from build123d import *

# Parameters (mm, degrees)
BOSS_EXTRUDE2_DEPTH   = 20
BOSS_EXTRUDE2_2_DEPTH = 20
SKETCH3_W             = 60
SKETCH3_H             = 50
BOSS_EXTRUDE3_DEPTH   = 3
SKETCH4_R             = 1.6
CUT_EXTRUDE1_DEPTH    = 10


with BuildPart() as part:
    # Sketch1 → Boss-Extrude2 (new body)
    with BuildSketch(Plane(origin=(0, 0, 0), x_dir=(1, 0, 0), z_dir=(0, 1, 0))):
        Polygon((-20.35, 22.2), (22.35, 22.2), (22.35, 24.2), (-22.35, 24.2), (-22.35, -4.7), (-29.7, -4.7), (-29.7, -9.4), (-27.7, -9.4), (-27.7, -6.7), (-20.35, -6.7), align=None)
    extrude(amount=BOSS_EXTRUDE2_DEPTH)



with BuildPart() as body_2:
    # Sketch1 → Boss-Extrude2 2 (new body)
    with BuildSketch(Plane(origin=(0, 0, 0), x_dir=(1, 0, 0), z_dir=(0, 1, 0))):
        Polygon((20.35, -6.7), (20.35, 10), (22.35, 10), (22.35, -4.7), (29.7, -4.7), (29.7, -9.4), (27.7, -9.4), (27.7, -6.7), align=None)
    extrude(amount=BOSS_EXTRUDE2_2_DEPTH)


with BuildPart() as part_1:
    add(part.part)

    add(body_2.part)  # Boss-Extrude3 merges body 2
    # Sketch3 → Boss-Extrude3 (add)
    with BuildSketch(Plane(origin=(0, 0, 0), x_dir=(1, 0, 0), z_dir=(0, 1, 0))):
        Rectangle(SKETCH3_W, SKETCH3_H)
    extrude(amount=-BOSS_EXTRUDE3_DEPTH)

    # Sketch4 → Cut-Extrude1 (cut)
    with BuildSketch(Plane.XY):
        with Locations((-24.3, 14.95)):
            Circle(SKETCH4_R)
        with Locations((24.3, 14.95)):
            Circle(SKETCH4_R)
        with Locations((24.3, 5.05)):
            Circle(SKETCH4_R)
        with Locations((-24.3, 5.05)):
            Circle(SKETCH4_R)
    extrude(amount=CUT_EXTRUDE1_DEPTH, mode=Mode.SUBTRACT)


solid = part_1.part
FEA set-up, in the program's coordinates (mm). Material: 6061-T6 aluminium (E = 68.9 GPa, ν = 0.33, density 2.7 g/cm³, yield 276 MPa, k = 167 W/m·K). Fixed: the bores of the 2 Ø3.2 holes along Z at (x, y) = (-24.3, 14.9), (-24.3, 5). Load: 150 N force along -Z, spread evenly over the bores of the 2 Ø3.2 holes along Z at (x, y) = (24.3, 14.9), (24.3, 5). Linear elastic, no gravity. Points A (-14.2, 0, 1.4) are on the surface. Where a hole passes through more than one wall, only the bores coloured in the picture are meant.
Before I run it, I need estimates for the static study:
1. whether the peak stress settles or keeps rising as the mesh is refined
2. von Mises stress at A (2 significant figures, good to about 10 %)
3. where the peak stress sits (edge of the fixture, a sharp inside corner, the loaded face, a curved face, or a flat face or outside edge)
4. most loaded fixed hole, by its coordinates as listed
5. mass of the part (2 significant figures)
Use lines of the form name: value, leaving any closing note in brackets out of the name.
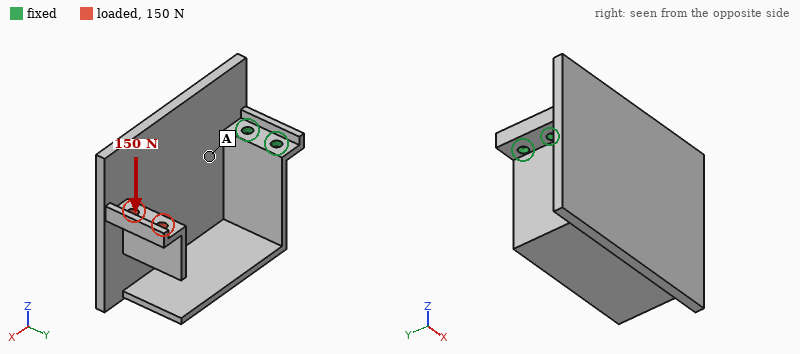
whether the peak stress settles or keeps rising as the mesh is refined: keeps rising
von Mises stress at A: 28 MPa
where the peak stress sits: edge of the fixture
most loaded fixed hole, by its coordinates as listed: (-24.3, 5)
mass of the part: 36 g
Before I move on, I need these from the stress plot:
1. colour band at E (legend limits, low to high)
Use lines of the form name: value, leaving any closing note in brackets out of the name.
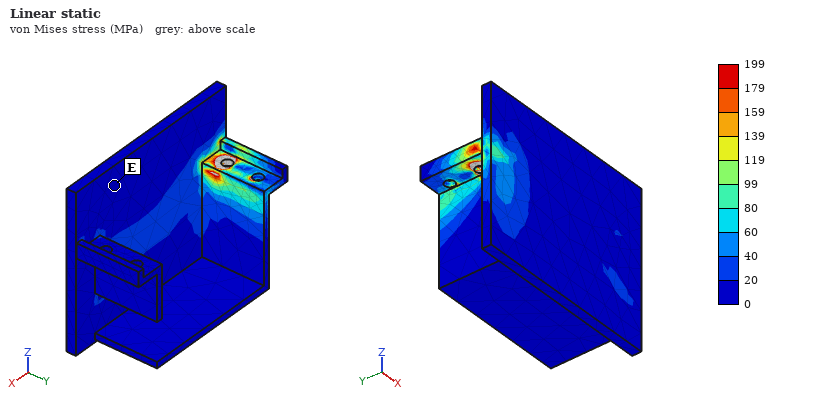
colour band at E: 0 to 20 MPa
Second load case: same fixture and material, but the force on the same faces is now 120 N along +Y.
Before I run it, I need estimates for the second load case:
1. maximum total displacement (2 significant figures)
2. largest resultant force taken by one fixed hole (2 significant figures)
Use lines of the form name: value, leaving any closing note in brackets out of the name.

maximum total displacement: 0.83 mm
largest resultant force taken by one fixed hole: 360 N
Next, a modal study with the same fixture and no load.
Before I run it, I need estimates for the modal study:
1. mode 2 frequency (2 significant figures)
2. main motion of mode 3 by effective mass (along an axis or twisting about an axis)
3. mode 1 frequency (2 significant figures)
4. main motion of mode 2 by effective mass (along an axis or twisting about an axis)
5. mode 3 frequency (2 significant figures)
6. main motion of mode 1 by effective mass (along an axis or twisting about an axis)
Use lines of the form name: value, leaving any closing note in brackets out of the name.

mode 2 frequency: 640 Hz
main motion of mode 3 by effective mass: twisting about X
mode 1 frequency: 550 Hz
main motion of mode 2 by effective mass: along Y
mode 3 frequency: 1500 Hz
main motion of mode 1 by effective mass: along Z
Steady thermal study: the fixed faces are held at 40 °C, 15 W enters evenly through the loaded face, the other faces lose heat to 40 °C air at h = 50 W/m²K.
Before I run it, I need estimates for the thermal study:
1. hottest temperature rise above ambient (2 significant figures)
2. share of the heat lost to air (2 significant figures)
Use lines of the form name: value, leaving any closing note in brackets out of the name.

hottest temperature rise above ambient: 49 K
share of the heat lost to air: 55 %
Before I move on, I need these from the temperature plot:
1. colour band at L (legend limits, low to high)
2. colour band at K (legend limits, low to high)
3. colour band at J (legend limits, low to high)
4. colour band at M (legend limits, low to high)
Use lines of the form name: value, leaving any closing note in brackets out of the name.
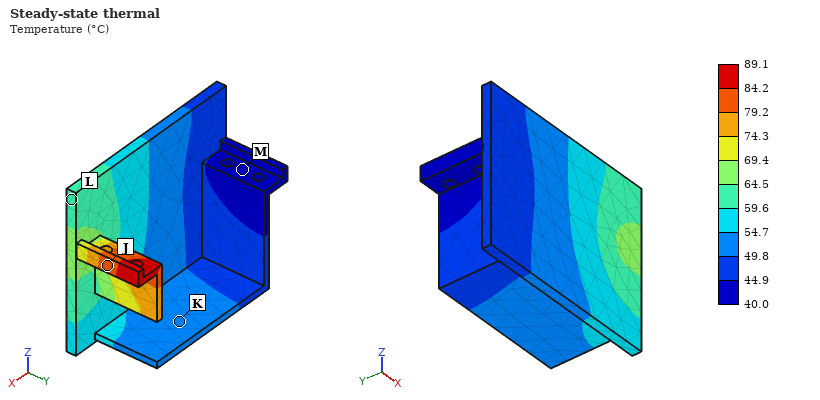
colour band at L: 59.6 to 64.5 °C
colour band at K: 49.8 to 54.7 °C
colour band at J: 79.2 to 84.2 °C
colour band at M: 40.0 to 44.9 °C
